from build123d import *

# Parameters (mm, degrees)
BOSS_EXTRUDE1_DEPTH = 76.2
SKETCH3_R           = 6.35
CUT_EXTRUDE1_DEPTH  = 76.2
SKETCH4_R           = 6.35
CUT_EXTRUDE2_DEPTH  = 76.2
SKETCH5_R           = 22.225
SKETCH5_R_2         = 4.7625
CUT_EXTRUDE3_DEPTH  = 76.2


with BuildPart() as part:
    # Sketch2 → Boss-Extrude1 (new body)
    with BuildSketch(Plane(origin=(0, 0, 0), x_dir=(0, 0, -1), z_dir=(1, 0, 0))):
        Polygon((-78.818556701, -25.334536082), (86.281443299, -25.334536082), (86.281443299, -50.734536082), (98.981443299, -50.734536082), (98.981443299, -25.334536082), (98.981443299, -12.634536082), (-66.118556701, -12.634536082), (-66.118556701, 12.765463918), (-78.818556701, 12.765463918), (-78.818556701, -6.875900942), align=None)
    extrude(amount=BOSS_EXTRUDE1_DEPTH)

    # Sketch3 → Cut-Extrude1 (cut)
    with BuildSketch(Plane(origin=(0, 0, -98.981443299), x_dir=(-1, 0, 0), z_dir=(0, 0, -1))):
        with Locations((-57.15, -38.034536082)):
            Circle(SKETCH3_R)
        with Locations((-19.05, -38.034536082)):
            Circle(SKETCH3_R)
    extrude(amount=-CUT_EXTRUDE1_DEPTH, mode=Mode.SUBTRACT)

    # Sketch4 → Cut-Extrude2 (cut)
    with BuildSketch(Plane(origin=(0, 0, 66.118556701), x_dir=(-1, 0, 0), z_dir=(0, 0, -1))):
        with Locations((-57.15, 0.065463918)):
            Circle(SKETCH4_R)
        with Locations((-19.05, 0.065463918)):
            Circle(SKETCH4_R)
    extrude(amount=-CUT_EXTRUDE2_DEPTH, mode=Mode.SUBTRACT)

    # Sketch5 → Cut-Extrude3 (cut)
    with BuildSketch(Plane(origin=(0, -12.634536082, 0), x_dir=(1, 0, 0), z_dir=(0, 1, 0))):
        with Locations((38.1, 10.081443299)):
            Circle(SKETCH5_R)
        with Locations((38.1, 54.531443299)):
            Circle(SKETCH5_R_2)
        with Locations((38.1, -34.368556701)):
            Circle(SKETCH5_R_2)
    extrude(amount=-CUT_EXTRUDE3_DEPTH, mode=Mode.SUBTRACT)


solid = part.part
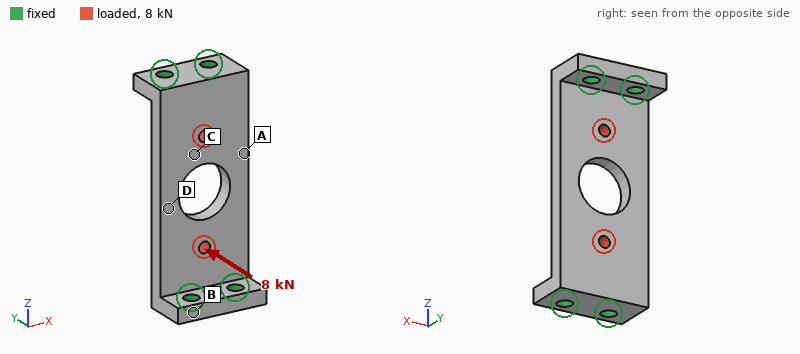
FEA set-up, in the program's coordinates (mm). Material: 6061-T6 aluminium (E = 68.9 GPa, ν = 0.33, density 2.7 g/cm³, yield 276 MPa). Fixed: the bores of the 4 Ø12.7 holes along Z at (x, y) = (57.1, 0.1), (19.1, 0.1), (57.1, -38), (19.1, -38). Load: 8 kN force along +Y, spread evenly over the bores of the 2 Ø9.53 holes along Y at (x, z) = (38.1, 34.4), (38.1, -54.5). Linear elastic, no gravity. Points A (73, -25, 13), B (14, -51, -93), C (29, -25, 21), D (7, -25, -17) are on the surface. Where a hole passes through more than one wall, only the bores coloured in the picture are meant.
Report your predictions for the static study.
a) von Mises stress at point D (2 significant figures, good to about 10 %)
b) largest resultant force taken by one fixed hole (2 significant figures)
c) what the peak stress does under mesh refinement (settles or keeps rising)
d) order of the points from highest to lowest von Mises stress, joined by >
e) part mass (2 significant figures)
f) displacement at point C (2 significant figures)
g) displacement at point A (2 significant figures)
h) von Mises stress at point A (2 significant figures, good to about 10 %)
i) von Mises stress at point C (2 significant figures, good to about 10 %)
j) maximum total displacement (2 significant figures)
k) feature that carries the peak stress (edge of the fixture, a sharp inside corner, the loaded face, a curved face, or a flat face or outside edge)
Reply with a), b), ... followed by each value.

a) 41 MPa
b) 2.1 kN
c) keeps rising
d) D > A > C > B
e) 520 g
f) 0.16 mm
g) 0.16 mm
h) 29 MPa
i) 17 MPa
j) 0.19 mm
k) edge of the fixture
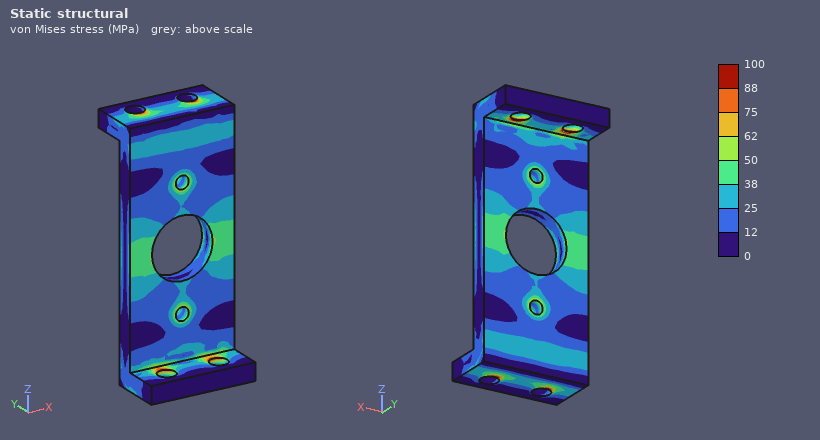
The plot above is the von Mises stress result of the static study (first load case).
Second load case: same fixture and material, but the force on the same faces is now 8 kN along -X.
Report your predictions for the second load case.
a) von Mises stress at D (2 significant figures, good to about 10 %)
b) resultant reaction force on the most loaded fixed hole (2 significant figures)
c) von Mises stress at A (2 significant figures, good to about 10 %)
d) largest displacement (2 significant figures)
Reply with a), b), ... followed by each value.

a) 7.1 MPa
b) 2.7 kN
c) 8.8 MPa
d) 19 µm
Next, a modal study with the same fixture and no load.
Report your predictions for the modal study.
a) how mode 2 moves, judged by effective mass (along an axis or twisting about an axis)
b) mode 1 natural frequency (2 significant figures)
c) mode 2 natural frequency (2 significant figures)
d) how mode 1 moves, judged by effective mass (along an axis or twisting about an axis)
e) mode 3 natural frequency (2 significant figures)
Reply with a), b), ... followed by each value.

a) twisting about Z
b) 2000 Hz
c) 3600 Hz
d) along Y
e) 5300 Hz
